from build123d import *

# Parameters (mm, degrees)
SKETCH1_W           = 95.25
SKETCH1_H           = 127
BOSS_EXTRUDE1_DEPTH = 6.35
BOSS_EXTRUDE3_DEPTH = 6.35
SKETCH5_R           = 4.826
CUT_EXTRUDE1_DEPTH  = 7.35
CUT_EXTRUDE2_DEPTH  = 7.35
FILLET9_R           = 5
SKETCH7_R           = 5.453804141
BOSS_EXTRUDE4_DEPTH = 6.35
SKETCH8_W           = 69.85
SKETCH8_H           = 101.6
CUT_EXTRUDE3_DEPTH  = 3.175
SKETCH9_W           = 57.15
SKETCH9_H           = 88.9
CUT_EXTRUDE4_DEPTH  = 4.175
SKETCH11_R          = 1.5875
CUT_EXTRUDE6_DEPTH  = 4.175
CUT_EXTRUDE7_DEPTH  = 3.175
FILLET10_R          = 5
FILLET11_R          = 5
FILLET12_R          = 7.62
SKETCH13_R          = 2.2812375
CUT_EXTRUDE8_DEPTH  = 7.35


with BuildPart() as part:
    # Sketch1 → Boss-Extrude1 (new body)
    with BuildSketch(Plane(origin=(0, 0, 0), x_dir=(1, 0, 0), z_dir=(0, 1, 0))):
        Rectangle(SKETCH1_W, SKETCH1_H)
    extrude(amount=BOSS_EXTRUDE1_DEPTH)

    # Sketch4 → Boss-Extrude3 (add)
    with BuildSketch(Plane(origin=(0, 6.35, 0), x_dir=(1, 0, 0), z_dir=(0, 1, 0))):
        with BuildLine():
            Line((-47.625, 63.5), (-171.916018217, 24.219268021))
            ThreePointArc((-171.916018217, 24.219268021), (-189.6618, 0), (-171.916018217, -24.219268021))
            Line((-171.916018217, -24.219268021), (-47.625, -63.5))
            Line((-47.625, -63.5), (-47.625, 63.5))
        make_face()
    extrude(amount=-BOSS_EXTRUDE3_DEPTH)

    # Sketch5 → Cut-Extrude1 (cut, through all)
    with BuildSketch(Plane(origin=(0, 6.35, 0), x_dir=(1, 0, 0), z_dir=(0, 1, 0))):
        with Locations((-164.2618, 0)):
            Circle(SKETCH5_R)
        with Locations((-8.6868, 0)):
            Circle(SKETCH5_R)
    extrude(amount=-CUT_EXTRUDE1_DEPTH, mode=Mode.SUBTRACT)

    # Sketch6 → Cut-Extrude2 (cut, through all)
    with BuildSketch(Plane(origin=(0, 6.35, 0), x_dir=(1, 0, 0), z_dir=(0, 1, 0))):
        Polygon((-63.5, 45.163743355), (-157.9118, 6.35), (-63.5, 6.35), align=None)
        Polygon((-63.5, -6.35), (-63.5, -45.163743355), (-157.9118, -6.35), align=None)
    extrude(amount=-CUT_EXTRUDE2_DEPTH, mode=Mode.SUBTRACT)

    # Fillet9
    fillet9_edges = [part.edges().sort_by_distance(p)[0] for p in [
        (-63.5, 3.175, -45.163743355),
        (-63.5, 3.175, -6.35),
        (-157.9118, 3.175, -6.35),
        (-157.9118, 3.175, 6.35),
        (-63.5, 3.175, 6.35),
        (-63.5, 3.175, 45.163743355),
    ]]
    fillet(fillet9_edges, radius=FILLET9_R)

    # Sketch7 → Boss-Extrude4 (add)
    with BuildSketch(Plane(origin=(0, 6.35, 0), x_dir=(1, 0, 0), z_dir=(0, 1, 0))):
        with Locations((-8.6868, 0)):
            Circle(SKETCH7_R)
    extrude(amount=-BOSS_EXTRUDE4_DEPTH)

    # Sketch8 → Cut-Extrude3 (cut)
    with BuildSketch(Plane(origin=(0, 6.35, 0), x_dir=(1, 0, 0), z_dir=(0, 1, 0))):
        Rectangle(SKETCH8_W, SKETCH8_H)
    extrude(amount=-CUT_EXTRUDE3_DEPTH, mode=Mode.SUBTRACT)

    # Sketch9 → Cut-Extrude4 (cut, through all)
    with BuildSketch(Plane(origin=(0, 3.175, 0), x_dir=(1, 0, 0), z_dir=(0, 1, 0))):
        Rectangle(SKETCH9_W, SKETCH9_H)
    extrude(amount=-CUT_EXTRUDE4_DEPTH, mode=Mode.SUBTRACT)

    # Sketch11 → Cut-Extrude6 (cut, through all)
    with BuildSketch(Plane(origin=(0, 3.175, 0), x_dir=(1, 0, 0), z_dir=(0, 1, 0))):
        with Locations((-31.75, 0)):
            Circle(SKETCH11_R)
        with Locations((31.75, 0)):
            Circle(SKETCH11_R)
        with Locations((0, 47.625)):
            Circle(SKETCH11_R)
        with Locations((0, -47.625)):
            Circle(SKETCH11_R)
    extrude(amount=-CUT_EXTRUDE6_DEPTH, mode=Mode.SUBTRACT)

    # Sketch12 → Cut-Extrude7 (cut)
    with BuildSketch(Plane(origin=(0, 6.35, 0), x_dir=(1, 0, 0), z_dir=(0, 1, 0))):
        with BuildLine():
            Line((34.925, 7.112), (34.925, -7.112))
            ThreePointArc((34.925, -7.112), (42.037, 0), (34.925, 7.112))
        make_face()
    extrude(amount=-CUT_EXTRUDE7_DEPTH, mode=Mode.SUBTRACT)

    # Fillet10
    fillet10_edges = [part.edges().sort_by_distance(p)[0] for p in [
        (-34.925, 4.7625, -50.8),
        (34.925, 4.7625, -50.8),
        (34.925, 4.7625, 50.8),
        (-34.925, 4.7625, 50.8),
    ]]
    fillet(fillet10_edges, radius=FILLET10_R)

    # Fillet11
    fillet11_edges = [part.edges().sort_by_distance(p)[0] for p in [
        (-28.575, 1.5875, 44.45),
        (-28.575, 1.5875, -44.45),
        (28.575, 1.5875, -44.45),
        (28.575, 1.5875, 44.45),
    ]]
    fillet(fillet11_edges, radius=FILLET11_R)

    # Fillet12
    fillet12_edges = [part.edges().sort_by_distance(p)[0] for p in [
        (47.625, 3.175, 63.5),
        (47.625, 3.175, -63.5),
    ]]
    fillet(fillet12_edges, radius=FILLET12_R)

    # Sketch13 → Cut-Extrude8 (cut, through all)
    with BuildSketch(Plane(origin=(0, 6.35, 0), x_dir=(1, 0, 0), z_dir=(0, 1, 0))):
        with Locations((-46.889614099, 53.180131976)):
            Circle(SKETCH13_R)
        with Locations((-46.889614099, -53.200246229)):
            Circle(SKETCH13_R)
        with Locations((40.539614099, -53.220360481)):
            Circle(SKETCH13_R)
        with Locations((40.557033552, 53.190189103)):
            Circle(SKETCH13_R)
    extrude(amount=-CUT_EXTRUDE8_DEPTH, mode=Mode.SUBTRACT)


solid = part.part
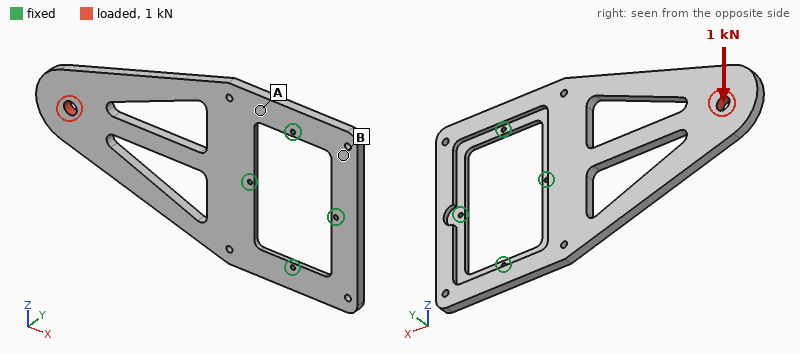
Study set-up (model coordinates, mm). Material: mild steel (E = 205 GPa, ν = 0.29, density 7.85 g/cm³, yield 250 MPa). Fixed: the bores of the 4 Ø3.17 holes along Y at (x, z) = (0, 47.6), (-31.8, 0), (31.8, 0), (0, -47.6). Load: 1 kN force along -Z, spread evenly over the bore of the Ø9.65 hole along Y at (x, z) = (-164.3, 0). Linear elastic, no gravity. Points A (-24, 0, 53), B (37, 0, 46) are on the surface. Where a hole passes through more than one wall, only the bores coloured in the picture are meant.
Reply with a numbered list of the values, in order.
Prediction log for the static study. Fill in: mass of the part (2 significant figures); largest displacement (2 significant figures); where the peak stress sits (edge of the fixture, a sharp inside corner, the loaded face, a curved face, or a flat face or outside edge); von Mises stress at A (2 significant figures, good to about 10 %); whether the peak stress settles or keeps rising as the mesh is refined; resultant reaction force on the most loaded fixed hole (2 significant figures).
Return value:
1. 690 g
2. 32 µm
3. edge of the fixture
4. 12 MPa
5. keeps rising
6. 1.2 kN
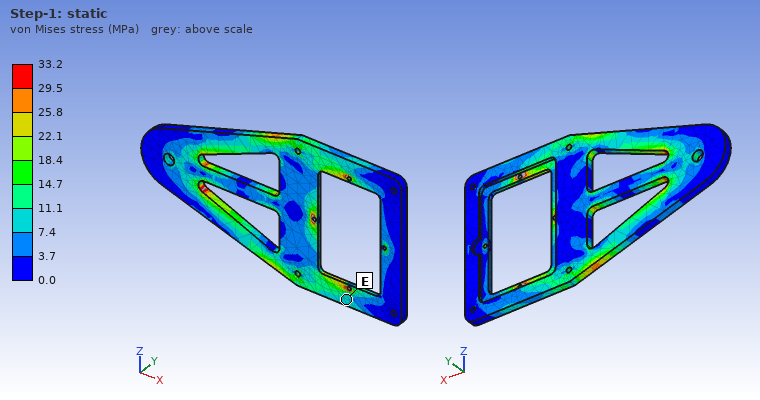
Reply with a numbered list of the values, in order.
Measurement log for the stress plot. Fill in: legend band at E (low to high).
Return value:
1. 7.4 to 11.1 MPa
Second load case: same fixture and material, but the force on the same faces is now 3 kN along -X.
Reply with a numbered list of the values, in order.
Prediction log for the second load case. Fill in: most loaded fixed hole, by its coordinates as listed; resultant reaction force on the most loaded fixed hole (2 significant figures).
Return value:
1. (-31.8, 0)
2. 1.2 kN
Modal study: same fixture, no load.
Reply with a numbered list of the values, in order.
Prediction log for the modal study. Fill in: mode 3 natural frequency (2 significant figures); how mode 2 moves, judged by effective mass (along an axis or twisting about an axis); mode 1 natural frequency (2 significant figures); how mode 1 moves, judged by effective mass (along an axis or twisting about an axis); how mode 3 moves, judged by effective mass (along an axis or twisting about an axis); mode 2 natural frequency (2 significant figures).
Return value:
1. 960 Hz
2. twisting about X
3. 170 Hz
4. along Y
5. along Y
6. 700 Hz
